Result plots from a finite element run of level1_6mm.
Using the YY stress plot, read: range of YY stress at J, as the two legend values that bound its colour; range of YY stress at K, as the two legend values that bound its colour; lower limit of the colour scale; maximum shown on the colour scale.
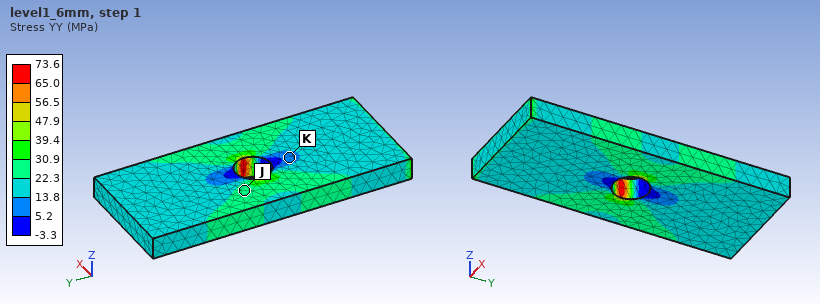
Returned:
22.3 to 30.9 MPa
5.2 to 13.8 MPa
-3.3 MPa
73.6 MPa
